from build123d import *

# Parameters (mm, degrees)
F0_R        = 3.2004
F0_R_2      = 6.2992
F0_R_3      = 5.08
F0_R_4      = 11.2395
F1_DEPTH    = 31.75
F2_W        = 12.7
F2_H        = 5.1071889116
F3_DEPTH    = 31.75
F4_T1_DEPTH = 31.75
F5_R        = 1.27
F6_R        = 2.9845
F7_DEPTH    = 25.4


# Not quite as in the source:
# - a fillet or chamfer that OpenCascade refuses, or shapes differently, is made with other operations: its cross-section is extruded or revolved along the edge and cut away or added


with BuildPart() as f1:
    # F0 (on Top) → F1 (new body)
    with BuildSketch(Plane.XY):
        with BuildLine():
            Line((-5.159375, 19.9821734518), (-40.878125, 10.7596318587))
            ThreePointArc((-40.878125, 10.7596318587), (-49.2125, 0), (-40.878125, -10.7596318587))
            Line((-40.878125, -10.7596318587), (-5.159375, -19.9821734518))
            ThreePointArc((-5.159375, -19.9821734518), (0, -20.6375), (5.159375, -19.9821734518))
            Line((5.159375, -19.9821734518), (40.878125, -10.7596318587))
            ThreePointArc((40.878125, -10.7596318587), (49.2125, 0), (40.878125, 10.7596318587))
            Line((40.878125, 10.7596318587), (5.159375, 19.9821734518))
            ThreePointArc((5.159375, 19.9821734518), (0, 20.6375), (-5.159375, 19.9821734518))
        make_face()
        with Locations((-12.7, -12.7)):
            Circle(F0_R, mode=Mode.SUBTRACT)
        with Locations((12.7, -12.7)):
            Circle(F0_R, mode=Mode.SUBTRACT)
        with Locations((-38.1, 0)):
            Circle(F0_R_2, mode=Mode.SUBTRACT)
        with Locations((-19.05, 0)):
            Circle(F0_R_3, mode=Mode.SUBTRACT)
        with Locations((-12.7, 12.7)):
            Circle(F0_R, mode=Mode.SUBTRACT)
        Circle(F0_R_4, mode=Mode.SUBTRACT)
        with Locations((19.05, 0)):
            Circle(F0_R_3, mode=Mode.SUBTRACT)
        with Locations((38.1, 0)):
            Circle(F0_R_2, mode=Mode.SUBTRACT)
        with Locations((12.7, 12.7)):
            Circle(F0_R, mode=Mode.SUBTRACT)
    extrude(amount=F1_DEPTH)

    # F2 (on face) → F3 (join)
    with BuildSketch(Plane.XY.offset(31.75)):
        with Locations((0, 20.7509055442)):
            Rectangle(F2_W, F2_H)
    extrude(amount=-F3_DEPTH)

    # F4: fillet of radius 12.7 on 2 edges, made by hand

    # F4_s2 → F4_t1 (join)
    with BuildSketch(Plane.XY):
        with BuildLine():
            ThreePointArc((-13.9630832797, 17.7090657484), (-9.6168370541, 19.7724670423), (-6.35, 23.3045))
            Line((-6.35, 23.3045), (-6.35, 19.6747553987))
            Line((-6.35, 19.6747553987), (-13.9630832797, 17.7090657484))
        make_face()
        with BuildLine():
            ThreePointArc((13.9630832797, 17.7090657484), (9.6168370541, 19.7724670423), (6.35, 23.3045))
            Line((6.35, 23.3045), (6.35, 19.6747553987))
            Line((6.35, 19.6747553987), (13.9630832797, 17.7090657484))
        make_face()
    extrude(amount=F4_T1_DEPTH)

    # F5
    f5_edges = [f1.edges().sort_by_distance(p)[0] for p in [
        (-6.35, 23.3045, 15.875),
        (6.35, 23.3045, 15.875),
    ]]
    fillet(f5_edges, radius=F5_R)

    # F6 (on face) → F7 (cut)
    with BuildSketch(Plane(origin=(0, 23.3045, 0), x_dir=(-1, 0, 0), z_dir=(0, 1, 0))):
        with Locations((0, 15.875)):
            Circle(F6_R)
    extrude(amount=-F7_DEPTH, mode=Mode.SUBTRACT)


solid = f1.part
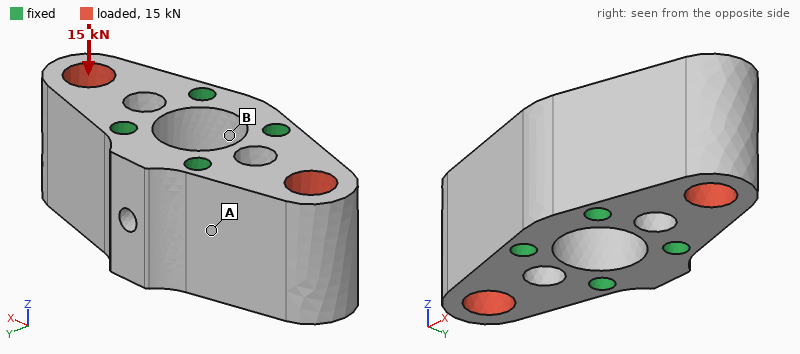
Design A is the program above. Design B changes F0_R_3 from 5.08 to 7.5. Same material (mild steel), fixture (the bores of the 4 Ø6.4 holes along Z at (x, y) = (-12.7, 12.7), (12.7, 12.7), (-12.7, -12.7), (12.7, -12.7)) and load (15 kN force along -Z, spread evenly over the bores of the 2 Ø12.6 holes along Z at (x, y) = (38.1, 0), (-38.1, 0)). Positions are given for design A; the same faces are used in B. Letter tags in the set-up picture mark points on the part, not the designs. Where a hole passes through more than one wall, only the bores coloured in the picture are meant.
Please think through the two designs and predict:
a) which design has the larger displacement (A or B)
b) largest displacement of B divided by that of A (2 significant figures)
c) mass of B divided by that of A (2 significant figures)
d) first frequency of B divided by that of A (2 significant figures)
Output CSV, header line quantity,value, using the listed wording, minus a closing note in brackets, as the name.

quantity,value
which design has the larger displacement,B
largest displacement of B divided by that of A,1.1
mass of B divided by that of A,0.90
first frequency of B divided by that of A,0.91
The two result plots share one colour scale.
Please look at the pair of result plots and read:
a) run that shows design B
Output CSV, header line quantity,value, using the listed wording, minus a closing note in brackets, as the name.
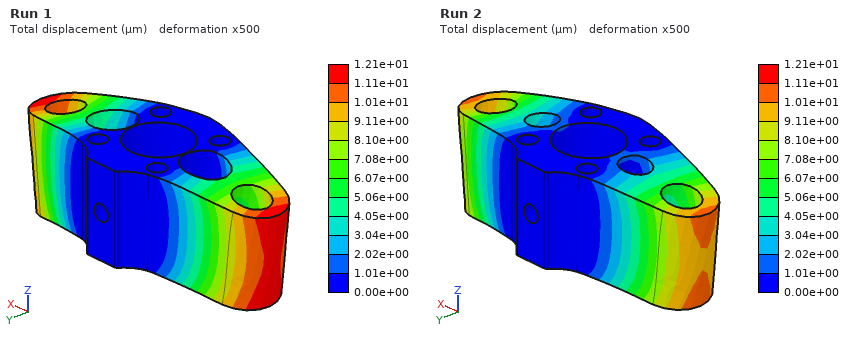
quantity,value
run that shows design B,Run 1
